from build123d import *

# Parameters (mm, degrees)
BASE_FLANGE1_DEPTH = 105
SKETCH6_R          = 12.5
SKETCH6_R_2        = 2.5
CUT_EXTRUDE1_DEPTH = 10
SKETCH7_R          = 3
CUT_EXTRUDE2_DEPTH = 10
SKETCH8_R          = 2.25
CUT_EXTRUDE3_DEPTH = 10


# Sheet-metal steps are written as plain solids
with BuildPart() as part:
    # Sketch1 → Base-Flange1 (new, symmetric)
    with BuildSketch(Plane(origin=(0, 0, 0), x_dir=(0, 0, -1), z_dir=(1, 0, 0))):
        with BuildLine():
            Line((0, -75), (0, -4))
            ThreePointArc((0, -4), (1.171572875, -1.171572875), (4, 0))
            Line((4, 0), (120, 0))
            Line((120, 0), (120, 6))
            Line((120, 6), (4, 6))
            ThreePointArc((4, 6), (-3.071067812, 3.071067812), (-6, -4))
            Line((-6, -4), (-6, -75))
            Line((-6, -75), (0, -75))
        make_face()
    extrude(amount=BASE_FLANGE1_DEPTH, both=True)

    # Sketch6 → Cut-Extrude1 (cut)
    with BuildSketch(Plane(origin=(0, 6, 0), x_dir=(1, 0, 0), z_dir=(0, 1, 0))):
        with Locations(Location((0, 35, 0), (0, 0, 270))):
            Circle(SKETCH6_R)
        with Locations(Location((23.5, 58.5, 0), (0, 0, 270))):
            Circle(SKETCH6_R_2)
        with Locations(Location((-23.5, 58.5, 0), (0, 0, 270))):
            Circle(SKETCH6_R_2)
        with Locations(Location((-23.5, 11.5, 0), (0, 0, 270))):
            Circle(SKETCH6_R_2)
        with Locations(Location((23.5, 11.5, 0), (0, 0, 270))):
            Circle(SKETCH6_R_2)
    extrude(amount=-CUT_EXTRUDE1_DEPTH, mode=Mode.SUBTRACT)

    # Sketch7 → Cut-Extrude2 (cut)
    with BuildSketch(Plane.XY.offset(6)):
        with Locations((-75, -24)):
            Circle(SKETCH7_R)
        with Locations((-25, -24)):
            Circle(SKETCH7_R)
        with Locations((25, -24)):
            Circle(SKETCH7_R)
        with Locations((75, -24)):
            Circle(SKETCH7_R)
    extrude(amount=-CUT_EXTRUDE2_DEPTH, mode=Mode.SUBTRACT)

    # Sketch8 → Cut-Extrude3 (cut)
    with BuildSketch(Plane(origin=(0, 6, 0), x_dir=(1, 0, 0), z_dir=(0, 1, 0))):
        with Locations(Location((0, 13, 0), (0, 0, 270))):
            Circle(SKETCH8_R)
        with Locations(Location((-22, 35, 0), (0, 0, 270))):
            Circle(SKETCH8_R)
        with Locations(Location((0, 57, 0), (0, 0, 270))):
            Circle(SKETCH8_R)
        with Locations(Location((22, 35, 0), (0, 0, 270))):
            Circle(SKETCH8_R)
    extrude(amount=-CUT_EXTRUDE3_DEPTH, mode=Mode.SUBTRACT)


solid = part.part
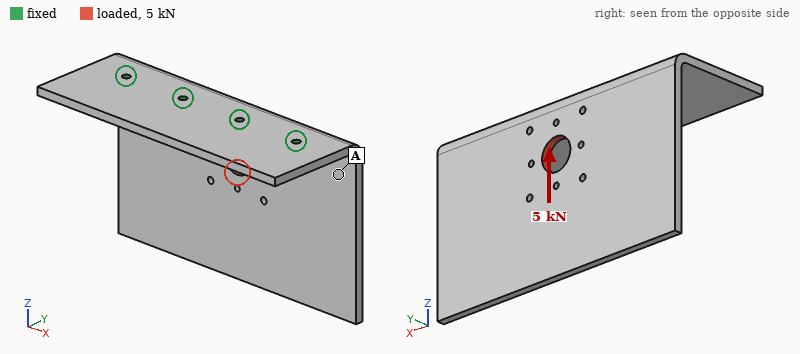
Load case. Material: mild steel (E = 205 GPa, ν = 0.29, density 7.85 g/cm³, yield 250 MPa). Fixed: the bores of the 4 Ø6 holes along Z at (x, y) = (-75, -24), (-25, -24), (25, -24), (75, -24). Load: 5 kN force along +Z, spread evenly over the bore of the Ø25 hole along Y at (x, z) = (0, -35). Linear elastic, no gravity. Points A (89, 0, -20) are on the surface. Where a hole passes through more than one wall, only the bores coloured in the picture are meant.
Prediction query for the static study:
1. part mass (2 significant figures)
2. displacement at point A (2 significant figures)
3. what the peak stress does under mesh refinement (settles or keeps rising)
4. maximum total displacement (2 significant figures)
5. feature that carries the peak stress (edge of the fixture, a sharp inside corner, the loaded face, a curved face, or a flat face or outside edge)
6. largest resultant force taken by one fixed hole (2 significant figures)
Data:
1.9 kg
0.081 mm
keeps rising
0.36 mm
edge of the fixture
1.3 kN
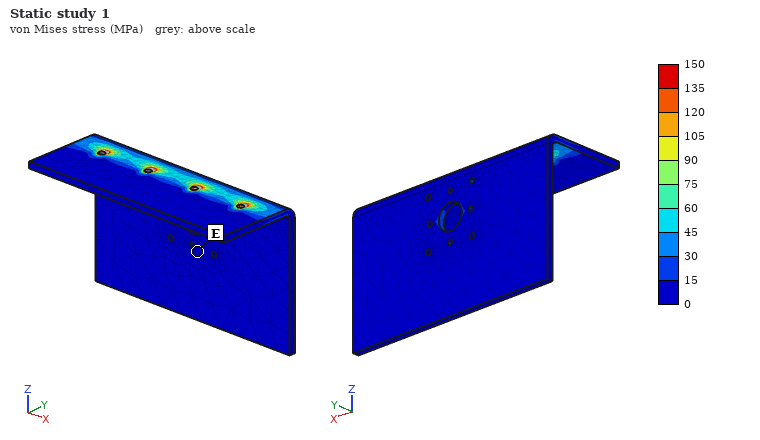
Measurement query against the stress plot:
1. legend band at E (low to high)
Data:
0 to 15 MPa
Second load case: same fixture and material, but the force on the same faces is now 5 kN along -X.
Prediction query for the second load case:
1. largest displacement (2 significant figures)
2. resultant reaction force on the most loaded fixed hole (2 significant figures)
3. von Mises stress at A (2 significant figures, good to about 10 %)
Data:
0.12 mm
1.8 kN
17 MPa
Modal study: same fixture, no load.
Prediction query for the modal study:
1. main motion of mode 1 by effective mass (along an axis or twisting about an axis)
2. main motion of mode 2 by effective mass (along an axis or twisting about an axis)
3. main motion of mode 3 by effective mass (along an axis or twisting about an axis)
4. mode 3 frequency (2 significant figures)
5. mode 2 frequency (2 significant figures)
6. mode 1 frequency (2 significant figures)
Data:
along Y
twisting about Z
along X
1100 Hz
460 Hz
240 Hz
